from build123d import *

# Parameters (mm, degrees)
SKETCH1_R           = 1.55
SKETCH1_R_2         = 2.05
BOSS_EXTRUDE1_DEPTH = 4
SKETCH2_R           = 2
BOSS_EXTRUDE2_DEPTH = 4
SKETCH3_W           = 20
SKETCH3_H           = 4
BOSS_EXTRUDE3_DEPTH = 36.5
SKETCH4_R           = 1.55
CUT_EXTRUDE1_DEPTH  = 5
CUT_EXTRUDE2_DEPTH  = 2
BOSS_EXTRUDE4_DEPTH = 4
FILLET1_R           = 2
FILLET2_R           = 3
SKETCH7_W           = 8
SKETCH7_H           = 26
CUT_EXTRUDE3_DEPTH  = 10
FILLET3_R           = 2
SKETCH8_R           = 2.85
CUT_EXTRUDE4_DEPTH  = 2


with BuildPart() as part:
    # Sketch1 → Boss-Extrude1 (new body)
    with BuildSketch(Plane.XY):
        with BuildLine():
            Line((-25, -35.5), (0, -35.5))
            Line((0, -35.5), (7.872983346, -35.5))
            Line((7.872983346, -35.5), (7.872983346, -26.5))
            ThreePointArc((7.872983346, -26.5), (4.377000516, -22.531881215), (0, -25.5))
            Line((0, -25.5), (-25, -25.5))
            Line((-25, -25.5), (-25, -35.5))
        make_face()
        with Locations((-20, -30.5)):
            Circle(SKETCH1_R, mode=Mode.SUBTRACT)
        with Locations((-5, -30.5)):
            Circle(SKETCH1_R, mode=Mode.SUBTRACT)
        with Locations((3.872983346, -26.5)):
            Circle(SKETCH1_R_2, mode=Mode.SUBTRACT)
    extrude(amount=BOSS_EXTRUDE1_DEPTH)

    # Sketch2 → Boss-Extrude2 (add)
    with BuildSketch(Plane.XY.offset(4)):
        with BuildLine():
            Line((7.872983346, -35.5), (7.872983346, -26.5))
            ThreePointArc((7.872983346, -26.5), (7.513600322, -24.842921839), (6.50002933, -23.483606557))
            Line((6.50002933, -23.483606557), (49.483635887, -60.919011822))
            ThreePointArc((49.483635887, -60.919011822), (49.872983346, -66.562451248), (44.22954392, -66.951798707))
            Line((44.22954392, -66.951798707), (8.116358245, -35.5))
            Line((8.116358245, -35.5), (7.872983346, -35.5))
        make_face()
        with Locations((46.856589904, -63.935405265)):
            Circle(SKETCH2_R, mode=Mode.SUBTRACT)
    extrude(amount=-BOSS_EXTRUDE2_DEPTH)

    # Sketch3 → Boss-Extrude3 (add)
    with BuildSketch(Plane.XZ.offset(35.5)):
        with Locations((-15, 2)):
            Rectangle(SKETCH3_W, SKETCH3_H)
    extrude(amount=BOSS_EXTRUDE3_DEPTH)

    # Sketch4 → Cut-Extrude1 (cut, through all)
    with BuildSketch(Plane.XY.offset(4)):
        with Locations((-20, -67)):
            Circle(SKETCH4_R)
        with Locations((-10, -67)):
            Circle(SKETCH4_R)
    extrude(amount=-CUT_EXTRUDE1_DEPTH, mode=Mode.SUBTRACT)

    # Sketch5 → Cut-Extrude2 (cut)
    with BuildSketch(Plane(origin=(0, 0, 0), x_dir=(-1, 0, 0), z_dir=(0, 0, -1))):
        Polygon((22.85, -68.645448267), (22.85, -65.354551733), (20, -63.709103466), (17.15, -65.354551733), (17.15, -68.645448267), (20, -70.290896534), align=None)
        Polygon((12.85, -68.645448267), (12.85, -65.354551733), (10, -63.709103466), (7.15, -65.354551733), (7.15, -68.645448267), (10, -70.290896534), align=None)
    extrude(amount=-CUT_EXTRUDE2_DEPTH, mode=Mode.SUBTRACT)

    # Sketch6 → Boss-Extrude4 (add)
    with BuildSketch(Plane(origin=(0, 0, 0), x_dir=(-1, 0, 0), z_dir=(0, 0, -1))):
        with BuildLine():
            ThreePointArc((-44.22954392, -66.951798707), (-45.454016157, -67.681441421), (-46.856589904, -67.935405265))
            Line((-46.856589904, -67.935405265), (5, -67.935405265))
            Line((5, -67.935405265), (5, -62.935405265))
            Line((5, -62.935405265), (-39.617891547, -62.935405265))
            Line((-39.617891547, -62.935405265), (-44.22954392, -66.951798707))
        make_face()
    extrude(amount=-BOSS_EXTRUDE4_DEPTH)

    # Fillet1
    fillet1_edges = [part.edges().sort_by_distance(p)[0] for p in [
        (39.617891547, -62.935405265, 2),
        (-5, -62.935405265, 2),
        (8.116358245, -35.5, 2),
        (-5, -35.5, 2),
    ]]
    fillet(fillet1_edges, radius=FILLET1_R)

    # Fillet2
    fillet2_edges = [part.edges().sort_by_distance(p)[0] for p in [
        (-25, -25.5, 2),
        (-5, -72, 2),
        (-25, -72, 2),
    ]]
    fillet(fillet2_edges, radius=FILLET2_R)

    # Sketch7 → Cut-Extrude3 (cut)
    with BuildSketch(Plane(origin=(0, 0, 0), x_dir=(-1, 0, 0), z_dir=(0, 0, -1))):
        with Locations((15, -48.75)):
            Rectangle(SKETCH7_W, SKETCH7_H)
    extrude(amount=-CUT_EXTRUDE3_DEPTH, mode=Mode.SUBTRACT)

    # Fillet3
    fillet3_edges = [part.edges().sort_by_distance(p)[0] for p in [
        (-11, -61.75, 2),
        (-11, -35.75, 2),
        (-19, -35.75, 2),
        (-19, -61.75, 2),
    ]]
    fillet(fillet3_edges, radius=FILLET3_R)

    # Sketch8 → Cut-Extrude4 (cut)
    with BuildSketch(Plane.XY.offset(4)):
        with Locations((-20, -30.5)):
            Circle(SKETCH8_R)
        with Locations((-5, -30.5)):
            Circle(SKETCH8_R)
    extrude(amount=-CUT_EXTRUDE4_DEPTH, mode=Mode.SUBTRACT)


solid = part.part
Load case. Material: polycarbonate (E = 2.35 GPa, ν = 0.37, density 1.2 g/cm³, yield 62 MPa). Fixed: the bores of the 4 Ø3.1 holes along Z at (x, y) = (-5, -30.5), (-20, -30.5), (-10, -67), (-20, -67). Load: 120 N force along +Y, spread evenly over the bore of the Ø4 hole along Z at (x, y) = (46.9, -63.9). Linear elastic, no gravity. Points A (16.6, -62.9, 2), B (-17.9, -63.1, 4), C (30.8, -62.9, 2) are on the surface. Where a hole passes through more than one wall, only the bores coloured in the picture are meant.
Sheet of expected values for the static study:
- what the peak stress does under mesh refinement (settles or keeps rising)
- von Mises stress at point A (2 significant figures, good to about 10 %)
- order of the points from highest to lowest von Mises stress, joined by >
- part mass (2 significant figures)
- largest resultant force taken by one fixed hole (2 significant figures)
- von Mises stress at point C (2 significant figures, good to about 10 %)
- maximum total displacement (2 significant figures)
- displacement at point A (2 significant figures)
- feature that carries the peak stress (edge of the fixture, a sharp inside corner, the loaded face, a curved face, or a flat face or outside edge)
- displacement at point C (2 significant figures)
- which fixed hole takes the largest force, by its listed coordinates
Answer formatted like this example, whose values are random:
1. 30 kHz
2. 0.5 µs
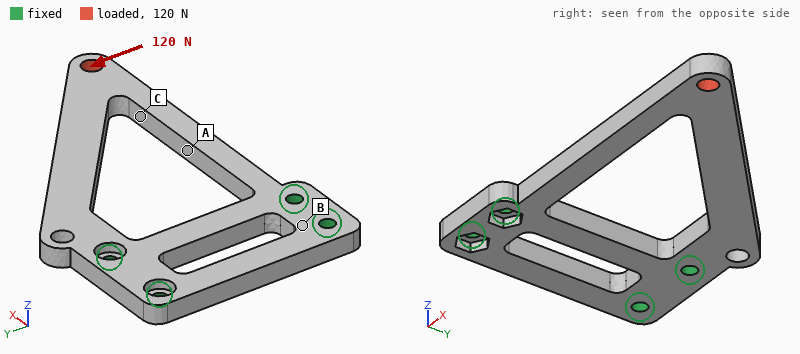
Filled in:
1. keeps rising
2. 7.2 MPa
3. C > A > B
4. 7.0 g
5. 200 N
6. 13 MPa
7. 0.80 mm
8. 0.35 mm
9. edge of the fixture
10. 0.61 mm
11. (-5, -30.5)
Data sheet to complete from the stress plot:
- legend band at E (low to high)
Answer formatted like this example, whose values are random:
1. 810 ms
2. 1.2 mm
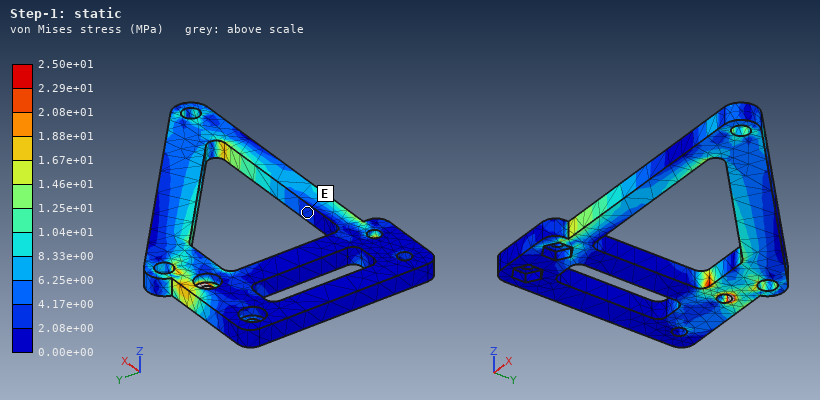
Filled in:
1. 2.08e+00 to 4.17e+00 MPa
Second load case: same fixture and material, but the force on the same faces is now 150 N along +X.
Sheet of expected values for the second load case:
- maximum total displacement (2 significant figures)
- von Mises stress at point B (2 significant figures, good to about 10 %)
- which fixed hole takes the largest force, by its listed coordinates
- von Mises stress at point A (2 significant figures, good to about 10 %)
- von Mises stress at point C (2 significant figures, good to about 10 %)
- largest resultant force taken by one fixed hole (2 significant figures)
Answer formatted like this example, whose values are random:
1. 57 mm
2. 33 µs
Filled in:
1. 0.32 mm
2. 1.2 MPa
3. (-10, -67)
4. 7.1 MPa
5. 8.8 MPa
6. 110 N
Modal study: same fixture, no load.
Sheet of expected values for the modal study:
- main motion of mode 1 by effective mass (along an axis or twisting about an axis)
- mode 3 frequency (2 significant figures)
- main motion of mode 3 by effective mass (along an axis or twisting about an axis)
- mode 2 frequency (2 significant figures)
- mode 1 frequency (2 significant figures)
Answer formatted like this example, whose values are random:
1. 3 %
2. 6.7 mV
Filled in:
1. along Z
2. 1300 Hz
3. along Y
4. 1100 Hz
5. 250 Hz
